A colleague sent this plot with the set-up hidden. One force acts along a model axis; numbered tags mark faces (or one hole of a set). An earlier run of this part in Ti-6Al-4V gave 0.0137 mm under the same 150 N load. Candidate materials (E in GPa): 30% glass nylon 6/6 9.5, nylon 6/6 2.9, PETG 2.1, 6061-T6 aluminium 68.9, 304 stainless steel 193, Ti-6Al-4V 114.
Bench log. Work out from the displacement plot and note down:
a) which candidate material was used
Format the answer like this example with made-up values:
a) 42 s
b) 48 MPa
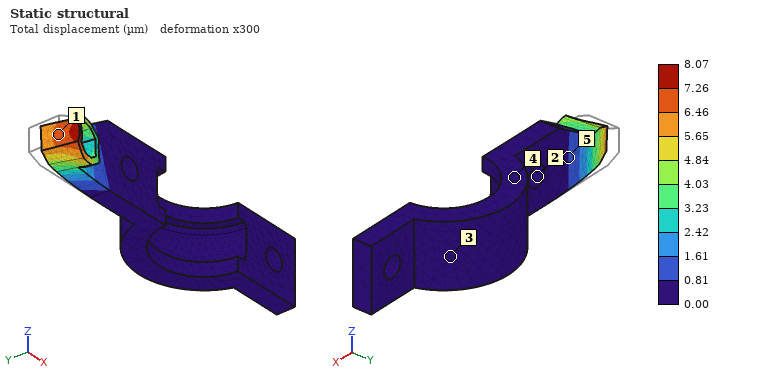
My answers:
a) 304 stainless steel
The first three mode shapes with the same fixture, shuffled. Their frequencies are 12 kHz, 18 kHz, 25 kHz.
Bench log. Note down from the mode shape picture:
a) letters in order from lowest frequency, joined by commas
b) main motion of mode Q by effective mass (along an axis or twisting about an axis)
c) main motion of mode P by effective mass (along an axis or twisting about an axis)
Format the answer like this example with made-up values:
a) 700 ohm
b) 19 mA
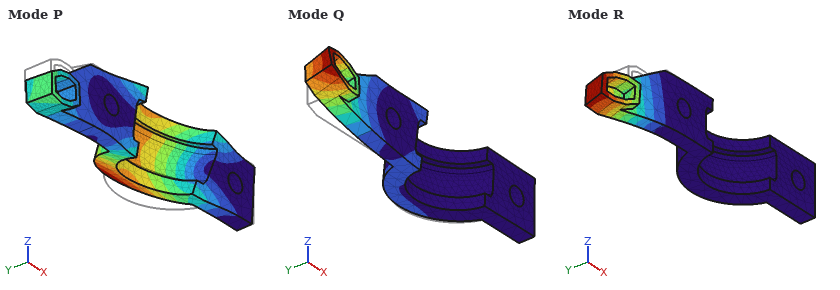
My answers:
a) R, P, Q
b) along Z
c) along Z
